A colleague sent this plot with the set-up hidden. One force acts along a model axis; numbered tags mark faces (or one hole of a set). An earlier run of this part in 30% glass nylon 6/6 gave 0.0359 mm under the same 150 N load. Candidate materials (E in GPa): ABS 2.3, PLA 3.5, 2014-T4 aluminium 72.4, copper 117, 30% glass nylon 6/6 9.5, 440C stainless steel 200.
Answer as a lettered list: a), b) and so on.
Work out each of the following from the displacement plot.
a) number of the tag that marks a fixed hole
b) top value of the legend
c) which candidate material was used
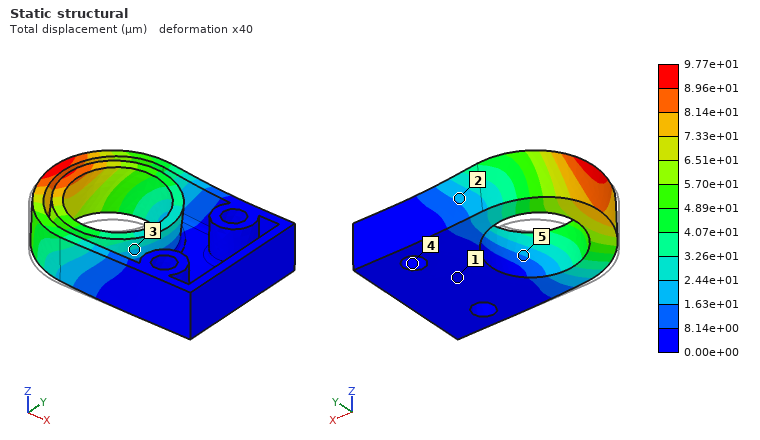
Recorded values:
a) 4
b) 9.77e+01 µm
c) PLA
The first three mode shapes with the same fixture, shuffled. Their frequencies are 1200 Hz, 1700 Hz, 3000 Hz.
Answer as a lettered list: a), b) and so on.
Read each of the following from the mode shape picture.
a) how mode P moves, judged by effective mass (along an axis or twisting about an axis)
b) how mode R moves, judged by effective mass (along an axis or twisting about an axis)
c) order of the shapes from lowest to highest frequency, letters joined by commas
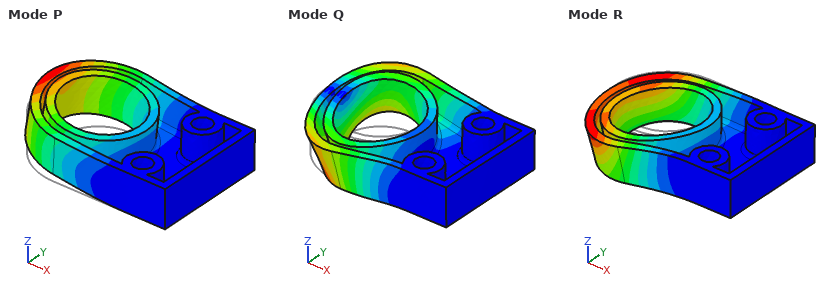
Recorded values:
a) along Z
b) along Y
c) P, R, Q
